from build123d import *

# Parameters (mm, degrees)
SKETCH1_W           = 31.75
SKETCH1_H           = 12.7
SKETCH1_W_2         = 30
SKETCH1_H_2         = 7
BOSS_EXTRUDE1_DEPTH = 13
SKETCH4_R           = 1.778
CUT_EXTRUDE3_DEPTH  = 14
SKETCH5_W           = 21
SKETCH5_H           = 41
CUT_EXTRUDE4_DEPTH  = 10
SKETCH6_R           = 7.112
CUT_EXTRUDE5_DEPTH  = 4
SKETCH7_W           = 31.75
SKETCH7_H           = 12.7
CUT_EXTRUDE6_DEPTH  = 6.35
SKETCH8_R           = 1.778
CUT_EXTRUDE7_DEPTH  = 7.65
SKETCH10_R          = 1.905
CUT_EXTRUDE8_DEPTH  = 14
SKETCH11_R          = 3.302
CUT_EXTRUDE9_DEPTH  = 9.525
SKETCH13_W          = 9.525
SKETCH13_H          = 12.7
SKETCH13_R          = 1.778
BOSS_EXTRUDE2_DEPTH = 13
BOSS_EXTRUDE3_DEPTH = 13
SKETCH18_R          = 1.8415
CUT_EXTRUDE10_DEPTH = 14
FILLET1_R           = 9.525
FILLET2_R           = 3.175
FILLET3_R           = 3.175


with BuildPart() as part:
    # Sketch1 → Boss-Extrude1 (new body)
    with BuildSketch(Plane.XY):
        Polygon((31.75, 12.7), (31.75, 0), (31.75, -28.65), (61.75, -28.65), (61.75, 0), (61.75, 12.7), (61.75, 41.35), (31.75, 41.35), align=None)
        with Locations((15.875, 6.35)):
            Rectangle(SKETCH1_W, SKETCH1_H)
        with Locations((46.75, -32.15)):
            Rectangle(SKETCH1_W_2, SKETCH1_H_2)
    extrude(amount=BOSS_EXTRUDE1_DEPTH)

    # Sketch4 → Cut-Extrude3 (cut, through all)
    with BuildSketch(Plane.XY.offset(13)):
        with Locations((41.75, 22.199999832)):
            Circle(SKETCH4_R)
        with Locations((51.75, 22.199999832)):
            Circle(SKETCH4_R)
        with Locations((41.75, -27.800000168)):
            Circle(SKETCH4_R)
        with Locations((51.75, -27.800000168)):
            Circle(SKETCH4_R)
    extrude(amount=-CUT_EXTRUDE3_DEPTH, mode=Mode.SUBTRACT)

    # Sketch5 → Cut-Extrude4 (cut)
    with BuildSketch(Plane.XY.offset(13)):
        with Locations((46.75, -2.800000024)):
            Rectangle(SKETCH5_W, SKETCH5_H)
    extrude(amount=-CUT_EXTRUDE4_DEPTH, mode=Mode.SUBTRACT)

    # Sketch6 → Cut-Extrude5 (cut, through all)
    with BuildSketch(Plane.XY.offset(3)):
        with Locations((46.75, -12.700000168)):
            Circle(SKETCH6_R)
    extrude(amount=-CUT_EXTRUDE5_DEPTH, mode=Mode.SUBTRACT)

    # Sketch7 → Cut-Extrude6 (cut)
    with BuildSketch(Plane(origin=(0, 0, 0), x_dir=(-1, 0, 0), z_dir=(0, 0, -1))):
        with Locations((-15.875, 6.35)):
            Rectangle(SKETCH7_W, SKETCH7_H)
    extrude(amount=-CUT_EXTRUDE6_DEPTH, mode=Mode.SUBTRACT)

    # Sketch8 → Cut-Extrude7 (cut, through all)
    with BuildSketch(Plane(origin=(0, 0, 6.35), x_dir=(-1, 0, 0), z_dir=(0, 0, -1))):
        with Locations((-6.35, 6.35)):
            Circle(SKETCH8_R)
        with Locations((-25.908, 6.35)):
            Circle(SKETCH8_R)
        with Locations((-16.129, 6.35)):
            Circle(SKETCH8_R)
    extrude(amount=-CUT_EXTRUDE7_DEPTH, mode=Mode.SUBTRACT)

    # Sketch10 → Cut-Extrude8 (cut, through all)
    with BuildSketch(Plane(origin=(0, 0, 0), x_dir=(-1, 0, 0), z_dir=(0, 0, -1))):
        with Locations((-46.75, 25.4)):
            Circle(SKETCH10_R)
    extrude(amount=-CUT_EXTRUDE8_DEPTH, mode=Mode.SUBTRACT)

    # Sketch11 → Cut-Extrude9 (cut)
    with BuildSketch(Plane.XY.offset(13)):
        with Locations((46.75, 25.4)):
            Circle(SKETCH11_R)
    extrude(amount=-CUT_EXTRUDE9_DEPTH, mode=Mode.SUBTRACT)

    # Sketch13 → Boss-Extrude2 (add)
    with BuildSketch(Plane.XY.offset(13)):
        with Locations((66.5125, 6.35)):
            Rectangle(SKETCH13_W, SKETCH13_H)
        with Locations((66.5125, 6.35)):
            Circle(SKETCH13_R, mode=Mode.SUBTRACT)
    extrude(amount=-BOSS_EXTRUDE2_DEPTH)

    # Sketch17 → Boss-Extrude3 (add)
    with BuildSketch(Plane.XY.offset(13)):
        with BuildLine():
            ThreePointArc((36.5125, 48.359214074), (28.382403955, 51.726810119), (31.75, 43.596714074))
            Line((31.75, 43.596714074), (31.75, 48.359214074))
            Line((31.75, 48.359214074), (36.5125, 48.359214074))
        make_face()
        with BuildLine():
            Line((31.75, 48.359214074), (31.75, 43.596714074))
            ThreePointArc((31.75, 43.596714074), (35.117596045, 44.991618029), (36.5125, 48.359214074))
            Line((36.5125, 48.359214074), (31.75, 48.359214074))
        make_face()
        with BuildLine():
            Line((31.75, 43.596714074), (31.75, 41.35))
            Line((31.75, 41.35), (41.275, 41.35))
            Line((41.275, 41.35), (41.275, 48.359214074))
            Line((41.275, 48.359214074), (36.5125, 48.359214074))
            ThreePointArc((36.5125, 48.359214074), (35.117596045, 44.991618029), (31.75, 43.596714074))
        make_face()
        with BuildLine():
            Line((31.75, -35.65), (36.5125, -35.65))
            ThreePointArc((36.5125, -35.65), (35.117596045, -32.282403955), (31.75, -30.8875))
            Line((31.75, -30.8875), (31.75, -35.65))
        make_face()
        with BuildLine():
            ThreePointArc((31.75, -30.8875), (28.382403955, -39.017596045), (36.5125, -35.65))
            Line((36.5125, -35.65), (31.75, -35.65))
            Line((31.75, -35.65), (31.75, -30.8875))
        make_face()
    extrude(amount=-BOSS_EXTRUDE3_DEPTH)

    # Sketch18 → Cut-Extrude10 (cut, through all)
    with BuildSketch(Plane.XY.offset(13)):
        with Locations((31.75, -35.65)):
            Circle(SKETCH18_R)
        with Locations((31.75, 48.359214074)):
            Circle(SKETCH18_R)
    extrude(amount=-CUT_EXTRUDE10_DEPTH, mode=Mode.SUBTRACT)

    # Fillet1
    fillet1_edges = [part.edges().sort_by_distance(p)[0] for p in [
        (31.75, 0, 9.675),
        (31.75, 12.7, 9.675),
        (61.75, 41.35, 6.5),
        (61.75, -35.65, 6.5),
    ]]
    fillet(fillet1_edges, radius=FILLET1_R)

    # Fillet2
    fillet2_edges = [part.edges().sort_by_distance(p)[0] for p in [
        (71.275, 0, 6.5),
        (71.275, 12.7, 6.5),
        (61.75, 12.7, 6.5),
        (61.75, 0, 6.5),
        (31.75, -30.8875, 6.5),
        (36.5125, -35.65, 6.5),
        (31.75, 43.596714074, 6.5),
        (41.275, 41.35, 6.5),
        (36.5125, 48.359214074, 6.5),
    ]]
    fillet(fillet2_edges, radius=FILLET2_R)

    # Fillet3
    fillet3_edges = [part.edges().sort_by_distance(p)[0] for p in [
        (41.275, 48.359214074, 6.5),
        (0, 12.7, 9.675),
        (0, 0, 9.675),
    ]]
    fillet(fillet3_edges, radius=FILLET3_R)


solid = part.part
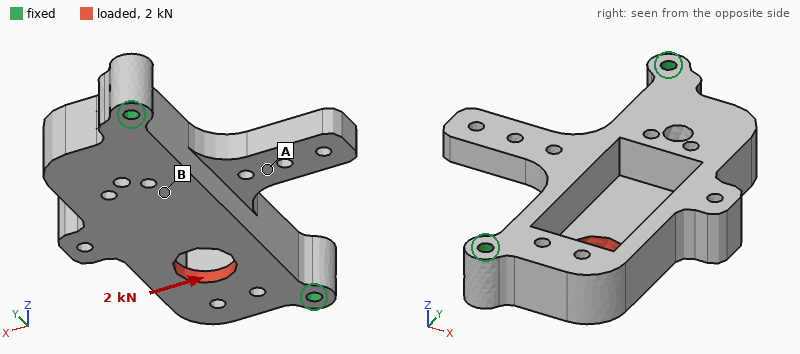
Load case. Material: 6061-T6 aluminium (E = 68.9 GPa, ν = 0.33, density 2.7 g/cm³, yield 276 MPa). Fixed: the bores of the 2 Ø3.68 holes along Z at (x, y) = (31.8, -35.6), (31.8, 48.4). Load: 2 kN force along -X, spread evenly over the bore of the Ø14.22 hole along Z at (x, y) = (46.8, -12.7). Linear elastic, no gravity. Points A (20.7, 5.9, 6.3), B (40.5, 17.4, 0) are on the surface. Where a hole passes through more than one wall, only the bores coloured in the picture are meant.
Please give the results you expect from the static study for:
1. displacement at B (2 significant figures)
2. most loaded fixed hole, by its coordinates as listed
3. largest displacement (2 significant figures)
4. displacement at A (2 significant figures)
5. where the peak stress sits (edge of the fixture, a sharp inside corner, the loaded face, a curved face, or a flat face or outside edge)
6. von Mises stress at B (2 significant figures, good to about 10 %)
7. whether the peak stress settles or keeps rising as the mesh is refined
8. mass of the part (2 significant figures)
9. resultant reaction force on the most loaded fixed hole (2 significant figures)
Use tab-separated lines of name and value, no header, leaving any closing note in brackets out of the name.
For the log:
displacement at B	15 µm
most loaded fixed hole, by its coordinates as listed	(31.8, -35.6)
largest displacement	36 µm
displacement at A	19 µm
where the peak stress sits	edge of the fixture
von Mises stress at B	11 MPa
whether the peak stress settles or keeps rising as the mesh is refined	keeps rising
mass of the part	70 g
resultant reaction force on the most loaded fixed hole	1.6 kN
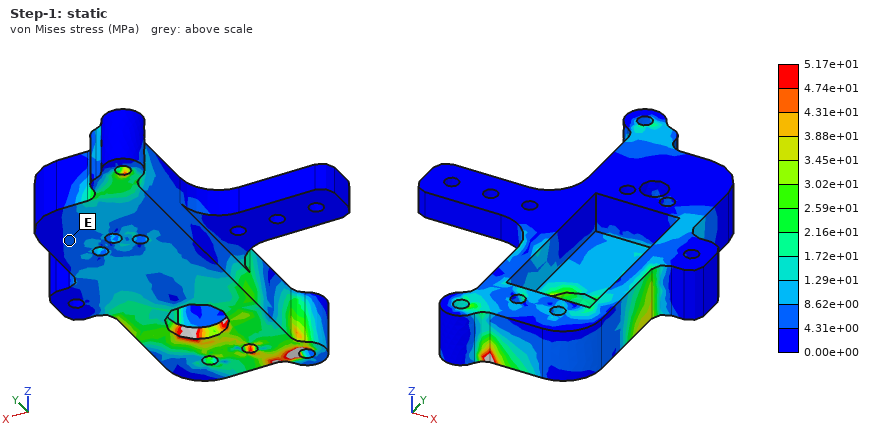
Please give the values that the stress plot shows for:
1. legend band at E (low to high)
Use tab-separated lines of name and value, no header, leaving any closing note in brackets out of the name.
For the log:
legend band at E	4.31e+00 to 8.62e+00 MPa
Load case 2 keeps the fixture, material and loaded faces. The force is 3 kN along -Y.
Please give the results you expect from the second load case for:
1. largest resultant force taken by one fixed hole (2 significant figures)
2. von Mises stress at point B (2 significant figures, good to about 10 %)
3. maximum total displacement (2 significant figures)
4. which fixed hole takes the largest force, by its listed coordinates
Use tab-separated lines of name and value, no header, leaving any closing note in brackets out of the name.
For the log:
largest resultant force taken by one fixed hole	1.7 kN
von Mises stress at point B	18 MPa
maximum total displacement	19 µm
which fixed hole takes the largest force, by its listed coordinates	(31.8, -35.6)
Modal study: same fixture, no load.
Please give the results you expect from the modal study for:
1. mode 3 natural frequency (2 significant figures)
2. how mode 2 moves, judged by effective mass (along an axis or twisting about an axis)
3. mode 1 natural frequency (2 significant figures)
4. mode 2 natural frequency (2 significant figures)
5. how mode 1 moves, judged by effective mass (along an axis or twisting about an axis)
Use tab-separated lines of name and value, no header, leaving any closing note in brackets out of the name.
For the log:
mode 3 natural frequency	6900 Hz
how mode 2 moves, judged by effective mass	along Z
mode 1 natural frequency	3000 Hz
mode 2 natural frequency	4100 Hz
how mode 1 moves, judged by effective mass	twisting about Y
